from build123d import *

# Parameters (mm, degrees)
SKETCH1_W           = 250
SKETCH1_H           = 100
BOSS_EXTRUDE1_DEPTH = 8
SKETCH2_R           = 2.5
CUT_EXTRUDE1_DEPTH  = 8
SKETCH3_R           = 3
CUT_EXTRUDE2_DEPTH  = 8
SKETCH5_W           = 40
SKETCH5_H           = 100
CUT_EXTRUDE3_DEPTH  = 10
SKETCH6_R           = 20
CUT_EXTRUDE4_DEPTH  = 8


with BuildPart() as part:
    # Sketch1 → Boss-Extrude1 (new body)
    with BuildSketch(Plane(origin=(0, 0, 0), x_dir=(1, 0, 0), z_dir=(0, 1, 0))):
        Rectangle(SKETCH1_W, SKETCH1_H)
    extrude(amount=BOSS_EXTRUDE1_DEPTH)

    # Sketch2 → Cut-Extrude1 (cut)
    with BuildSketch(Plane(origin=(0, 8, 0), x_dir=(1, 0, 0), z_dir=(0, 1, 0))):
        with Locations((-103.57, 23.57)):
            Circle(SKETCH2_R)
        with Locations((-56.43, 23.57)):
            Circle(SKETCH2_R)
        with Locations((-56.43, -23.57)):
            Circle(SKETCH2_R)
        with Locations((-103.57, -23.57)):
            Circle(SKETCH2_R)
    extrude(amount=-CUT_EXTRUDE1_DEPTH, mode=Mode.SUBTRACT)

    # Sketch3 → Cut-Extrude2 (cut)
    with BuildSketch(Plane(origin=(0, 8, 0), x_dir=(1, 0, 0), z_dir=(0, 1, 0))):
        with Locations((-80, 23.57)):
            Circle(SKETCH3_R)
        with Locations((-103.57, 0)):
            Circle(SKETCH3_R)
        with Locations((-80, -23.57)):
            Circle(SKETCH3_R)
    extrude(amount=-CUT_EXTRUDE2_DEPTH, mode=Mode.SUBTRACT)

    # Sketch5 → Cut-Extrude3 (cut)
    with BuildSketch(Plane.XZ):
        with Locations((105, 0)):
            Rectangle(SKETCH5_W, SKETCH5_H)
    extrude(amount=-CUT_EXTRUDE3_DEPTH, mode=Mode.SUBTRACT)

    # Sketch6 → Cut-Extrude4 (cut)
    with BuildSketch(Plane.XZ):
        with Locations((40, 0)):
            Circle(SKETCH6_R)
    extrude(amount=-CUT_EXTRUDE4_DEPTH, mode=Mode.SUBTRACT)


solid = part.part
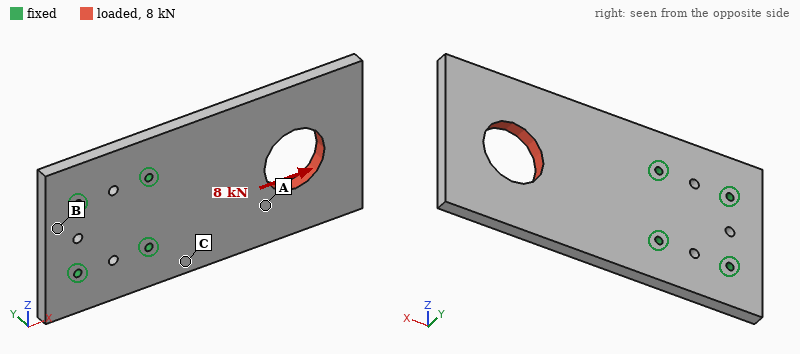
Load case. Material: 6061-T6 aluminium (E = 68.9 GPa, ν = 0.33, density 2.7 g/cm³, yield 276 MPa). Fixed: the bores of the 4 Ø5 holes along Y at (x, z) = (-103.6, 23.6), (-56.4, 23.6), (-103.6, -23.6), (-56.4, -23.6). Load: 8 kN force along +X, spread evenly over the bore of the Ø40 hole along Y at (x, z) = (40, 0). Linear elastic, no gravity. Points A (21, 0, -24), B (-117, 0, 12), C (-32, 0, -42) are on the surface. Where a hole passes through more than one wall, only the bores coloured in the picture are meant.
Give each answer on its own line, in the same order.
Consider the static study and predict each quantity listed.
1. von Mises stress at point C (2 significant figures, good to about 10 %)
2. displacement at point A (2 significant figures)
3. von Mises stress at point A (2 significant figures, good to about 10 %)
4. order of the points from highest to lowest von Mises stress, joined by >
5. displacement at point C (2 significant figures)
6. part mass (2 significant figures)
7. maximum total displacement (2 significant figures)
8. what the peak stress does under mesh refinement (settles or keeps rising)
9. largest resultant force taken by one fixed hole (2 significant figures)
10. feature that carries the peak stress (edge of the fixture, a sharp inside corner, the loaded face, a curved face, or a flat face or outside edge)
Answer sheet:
9.2 MPa
15 µm
16 MPa
A > C > B
6.8 µm
420 g
28 µm
keeps rising
3.1 kN
edge of the fixture
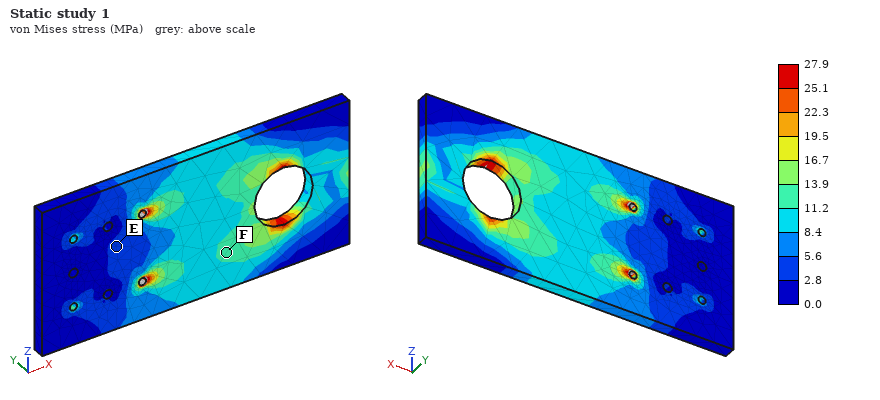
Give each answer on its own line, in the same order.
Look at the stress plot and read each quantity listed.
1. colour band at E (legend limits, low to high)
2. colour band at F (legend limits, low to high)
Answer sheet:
2.8 to 5.6 MPa
11.2 to 13.9 MPa
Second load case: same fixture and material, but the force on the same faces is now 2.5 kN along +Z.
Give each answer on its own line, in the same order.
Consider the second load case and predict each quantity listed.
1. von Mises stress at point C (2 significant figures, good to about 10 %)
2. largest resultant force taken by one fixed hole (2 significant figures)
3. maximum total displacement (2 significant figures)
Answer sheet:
10 MPa
3.4 kN
71 µm
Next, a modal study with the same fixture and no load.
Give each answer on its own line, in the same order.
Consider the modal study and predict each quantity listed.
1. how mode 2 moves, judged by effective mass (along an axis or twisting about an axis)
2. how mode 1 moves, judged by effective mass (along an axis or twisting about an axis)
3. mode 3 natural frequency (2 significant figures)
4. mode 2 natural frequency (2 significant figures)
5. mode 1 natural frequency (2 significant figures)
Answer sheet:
twisting about X
along Y
1800 Hz
940 Hz
330 Hz
